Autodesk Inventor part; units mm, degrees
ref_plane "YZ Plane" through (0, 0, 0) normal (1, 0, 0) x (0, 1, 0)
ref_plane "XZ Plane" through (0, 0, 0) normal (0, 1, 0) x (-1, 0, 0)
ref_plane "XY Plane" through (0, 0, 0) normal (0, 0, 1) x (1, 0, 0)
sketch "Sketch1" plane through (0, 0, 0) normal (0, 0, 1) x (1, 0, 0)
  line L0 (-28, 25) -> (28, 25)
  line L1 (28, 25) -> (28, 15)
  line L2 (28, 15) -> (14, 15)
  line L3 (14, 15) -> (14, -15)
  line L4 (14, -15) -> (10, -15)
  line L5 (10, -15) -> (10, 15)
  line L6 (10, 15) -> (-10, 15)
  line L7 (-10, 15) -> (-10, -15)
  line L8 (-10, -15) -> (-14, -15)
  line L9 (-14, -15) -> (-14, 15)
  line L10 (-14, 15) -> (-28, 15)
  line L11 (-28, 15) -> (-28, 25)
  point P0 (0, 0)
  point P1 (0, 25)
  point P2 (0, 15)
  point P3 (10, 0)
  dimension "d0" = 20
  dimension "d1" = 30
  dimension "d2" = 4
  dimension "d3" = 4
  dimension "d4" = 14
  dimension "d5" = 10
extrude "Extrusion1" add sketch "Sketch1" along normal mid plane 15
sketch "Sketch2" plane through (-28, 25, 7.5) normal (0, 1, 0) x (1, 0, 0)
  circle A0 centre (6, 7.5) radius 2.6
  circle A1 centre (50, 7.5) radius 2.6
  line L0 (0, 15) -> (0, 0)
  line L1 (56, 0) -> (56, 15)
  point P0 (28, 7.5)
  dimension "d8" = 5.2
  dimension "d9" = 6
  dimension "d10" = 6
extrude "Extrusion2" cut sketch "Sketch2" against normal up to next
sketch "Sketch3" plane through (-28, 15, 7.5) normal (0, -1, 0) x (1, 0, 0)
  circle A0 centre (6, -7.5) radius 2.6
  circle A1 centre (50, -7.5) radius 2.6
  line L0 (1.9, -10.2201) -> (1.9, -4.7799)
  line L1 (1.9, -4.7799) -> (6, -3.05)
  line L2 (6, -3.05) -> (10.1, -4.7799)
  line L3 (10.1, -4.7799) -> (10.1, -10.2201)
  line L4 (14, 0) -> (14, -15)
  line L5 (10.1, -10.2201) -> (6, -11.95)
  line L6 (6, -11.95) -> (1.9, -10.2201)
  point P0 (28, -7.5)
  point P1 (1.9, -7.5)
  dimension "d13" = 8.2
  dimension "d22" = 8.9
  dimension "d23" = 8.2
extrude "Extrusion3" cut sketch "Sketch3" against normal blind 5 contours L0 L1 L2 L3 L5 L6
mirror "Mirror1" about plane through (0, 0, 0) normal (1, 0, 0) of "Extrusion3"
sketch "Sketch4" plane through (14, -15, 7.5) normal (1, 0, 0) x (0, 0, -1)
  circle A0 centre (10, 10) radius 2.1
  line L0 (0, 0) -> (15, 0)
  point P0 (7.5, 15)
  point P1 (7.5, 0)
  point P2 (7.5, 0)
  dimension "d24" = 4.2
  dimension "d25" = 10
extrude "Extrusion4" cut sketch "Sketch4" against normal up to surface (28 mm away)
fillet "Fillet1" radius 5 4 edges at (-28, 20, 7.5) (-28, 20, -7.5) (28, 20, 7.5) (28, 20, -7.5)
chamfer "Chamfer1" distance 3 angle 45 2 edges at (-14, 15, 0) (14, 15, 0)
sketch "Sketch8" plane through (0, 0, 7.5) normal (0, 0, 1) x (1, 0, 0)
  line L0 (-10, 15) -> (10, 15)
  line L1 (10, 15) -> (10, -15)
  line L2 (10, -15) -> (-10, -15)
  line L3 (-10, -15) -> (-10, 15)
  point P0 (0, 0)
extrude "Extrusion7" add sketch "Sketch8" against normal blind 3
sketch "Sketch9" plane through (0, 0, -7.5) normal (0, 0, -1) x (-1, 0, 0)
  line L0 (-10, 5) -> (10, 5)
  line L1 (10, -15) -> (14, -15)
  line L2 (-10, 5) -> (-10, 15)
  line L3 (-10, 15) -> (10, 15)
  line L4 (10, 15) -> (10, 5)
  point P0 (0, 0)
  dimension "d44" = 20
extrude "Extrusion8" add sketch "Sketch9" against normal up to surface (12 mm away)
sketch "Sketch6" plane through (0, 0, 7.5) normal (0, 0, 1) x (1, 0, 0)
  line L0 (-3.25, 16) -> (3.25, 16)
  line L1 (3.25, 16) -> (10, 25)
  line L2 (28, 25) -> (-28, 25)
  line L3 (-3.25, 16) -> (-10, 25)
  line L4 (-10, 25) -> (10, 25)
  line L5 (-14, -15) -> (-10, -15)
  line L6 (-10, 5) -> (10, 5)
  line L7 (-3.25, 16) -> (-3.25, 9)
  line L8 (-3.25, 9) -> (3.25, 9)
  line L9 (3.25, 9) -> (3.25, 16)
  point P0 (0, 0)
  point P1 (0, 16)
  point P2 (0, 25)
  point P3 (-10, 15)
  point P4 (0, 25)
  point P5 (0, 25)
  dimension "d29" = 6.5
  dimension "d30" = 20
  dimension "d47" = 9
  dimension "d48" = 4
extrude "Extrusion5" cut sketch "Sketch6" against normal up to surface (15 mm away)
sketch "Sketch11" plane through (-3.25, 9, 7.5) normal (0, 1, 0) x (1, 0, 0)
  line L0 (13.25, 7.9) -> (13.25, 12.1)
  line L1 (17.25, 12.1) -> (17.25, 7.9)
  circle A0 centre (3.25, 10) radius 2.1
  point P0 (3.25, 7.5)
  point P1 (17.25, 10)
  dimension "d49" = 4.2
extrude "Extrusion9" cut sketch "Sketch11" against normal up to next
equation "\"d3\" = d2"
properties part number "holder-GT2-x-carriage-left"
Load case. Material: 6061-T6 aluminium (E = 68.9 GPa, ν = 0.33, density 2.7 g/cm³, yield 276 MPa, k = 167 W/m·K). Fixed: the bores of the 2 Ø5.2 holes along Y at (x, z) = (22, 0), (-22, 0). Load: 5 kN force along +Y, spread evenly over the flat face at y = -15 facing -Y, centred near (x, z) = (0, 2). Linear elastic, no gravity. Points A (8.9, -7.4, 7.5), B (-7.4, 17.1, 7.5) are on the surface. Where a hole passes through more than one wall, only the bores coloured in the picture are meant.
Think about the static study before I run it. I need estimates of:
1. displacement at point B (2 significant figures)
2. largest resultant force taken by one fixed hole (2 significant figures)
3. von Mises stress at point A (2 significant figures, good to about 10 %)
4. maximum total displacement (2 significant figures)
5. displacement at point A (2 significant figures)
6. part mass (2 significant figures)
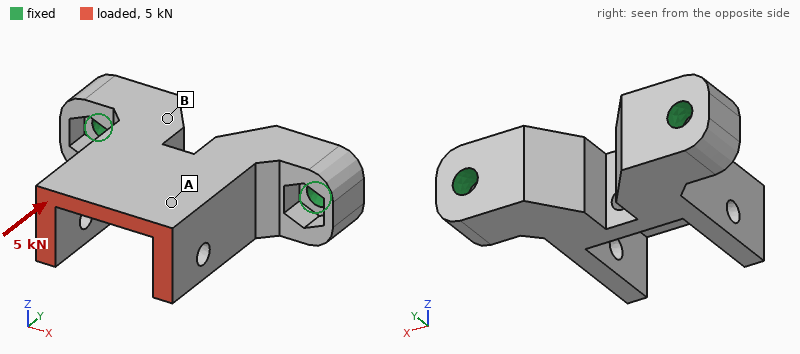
26 µm
2.9 kN
26 MPa
57 µm
49 µm
34 g
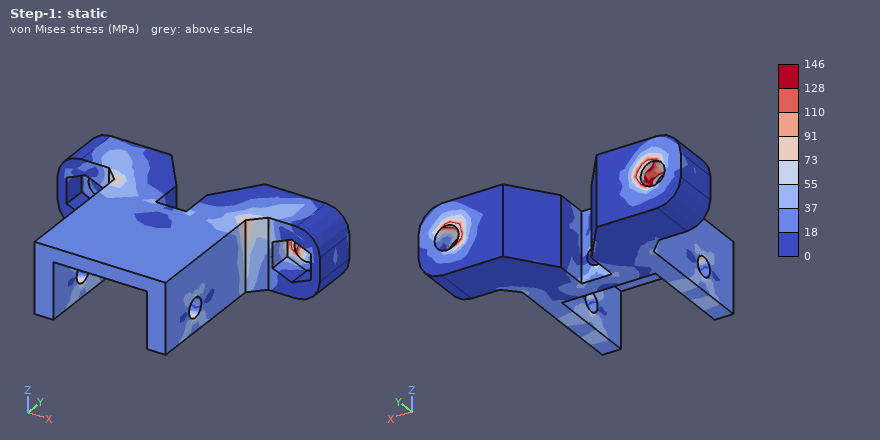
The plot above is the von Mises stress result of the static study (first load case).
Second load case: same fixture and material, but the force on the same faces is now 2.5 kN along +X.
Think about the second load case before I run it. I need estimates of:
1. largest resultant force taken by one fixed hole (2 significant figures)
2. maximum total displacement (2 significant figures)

2.7 kN
0.24 mm
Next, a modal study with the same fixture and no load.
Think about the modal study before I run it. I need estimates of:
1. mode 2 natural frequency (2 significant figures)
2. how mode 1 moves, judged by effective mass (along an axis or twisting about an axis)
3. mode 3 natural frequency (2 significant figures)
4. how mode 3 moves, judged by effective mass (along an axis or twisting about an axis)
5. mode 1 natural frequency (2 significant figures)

8300 Hz
along Z
13 kHz
along X
4500 Hz
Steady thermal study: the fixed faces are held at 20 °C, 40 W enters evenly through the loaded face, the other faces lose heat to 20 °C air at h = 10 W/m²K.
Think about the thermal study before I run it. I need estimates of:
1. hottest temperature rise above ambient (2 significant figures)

49 K
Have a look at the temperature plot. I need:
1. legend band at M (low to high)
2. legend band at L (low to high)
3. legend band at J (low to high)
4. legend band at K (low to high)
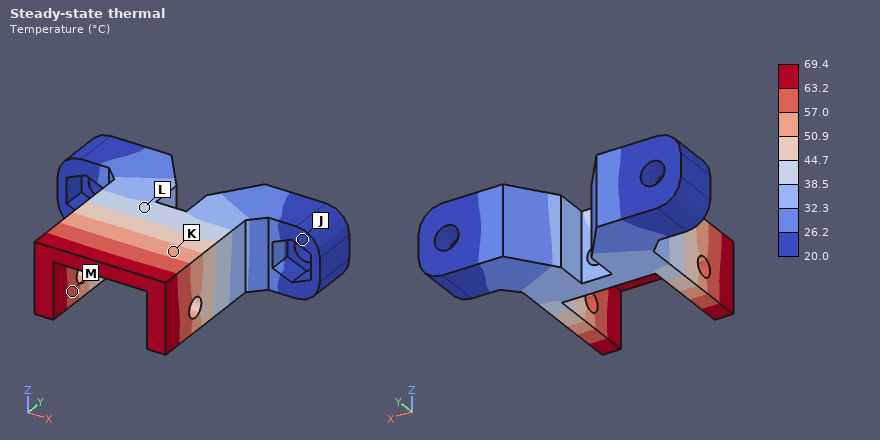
57.0 to 63.2 °C
38.5 to 44.7 °C
20.0 to 26.2 °C
50.9 to 57.0 °C
